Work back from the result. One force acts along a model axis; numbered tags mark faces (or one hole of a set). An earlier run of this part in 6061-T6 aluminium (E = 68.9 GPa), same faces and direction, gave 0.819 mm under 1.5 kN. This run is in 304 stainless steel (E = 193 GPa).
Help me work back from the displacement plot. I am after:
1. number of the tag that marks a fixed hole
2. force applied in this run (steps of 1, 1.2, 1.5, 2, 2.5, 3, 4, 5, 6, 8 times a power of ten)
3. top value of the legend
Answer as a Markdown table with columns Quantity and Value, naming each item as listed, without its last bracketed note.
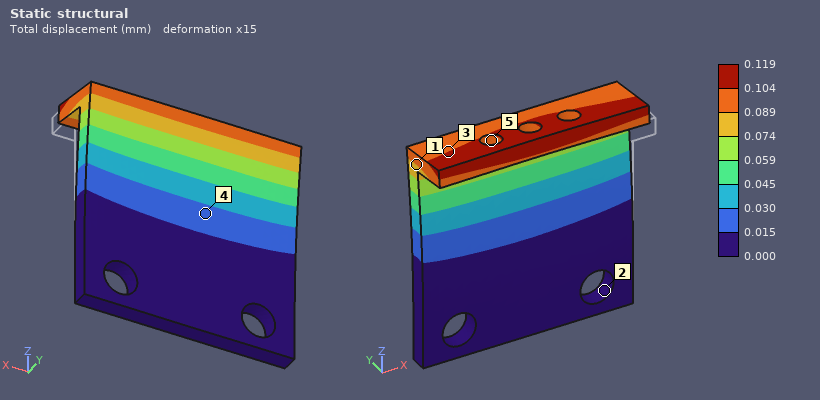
| Quantity | Value |
|---|---|
| number of the tag that marks a fixed hole | 2 |
| force applied in this run | 600 N |
| top value of the legend | 0.119 mm |
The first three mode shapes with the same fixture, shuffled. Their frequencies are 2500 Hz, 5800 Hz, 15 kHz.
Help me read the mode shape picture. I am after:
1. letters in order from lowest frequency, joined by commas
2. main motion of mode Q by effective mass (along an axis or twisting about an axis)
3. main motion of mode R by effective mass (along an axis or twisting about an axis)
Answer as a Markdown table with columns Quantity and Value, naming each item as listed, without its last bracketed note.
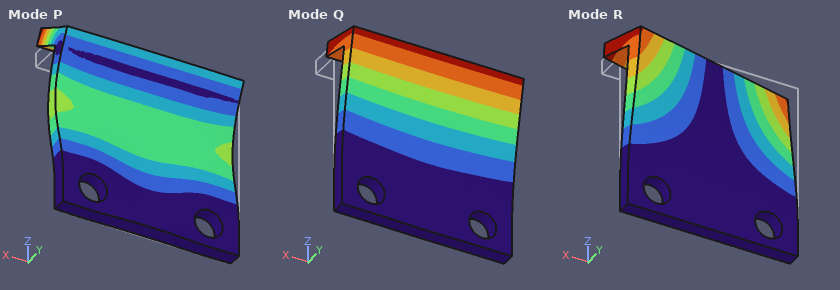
| Quantity | Value |
|---|---|
| letters in order from lowest frequency, joined by commas | Q, R, P |
| main motion of mode Q by effective mass | along Y |
| main motion of mode R by effective mass | twisting about Z |
